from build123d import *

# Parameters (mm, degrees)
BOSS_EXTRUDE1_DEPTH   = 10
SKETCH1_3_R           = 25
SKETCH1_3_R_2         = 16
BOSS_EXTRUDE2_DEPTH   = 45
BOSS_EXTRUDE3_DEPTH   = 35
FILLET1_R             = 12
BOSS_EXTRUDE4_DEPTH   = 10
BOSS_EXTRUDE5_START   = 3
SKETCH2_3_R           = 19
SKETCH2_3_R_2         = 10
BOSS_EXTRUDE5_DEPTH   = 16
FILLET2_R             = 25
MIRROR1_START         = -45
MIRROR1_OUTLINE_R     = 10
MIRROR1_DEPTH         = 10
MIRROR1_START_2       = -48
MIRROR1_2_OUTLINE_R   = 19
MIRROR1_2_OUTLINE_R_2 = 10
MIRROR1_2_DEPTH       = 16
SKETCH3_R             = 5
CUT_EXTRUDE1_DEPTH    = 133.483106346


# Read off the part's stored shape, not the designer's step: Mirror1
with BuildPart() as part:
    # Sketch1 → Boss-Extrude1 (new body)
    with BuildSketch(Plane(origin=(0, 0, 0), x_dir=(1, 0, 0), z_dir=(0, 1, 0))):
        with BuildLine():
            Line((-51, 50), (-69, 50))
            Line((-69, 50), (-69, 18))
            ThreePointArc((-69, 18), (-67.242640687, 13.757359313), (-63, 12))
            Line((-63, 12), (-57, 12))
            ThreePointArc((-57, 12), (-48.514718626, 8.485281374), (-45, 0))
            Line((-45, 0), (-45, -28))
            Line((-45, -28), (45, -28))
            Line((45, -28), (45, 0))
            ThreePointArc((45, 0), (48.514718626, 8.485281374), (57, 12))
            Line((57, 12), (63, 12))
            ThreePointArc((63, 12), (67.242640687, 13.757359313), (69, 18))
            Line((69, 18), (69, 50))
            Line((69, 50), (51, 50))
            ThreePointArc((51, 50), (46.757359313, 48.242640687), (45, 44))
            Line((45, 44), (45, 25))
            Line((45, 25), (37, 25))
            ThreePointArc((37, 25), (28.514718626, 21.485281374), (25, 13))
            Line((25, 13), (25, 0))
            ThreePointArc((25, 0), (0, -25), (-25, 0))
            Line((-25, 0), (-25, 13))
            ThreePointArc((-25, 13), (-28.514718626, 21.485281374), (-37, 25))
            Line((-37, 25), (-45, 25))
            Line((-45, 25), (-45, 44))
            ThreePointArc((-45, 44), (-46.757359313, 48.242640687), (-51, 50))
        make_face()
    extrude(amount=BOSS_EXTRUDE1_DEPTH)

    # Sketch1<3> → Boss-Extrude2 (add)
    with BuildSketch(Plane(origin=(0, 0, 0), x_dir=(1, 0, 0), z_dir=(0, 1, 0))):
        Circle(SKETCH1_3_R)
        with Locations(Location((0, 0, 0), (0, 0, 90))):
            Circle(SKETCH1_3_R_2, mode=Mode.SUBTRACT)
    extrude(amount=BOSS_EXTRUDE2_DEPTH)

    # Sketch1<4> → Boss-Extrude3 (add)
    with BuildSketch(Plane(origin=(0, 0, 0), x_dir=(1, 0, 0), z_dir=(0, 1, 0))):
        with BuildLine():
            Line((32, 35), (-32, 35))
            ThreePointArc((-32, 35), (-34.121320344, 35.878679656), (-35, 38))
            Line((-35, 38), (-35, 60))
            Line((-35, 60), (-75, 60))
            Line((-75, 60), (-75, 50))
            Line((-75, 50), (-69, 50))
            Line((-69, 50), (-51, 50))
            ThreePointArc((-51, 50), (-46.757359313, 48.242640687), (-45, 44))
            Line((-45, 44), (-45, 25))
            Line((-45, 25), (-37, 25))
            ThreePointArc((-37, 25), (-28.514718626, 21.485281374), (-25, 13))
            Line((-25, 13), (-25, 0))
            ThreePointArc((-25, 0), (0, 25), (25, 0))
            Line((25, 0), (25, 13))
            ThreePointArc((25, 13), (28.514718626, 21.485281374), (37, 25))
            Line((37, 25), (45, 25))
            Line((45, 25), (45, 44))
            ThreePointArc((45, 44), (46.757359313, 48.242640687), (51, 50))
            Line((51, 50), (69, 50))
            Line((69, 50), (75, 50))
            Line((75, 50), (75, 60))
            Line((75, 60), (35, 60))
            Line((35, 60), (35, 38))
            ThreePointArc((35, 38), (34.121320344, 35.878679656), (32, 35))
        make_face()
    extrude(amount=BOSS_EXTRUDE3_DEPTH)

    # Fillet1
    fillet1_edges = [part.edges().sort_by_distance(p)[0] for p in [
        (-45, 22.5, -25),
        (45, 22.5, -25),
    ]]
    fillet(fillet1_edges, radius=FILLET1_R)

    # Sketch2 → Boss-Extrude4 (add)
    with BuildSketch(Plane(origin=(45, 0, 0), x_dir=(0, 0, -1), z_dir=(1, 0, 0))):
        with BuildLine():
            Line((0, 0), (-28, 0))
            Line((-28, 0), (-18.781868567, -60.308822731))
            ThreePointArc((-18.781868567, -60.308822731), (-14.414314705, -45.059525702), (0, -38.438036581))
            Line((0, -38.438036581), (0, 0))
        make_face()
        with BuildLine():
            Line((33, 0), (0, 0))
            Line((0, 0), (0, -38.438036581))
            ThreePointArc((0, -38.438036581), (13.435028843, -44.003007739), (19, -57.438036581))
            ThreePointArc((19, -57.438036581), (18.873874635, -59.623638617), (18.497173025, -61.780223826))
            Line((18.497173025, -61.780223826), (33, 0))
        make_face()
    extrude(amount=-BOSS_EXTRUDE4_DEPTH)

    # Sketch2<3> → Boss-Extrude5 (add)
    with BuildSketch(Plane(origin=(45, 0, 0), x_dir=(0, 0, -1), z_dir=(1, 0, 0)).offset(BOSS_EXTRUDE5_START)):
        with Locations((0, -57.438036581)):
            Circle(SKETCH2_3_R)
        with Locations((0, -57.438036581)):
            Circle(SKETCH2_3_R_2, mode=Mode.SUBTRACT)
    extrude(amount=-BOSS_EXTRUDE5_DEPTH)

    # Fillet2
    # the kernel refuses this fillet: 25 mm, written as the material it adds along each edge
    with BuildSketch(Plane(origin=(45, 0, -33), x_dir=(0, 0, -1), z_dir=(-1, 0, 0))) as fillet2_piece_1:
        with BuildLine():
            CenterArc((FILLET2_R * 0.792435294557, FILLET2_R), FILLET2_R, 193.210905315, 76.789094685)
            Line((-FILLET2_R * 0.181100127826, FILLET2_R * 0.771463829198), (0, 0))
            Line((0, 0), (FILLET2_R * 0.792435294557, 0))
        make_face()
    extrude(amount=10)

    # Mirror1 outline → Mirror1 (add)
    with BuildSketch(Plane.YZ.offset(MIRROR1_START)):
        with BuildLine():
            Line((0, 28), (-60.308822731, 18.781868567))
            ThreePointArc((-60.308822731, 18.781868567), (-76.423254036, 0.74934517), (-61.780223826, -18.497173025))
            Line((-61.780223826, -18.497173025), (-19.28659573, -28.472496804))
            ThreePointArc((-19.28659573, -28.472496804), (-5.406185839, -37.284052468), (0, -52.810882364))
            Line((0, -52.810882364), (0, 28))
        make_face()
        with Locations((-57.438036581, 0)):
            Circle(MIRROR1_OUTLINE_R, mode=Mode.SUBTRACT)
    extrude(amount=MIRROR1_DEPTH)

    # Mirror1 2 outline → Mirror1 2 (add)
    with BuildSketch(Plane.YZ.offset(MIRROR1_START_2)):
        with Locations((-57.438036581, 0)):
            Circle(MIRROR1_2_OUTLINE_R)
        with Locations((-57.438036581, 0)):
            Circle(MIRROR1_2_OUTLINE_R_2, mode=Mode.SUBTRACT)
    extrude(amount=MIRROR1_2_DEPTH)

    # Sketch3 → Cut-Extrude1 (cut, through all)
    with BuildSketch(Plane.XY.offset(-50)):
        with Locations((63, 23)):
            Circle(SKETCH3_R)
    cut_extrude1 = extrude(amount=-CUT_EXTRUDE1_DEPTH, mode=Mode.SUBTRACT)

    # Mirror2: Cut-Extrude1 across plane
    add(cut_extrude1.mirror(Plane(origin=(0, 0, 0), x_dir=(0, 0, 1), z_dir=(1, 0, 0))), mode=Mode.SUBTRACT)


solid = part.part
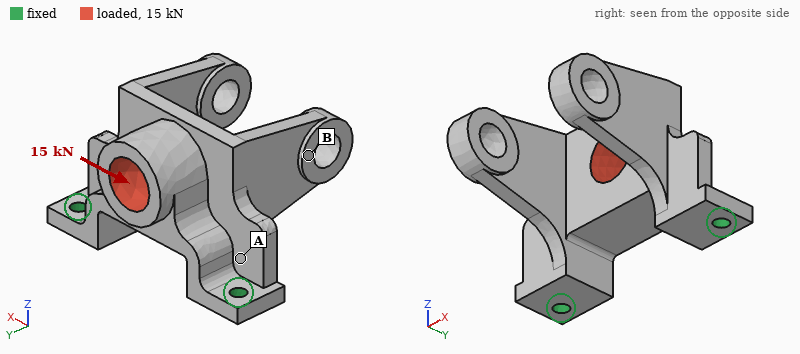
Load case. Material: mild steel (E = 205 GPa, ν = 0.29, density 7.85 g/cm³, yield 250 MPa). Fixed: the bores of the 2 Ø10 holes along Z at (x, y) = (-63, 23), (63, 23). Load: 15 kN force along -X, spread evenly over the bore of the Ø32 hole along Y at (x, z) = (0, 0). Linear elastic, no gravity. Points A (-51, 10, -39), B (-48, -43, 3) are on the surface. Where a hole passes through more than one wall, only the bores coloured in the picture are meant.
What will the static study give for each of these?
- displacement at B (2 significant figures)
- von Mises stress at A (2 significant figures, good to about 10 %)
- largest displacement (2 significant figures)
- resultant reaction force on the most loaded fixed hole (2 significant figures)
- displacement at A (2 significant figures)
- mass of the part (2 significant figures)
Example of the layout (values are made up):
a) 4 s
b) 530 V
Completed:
a) 22 µm
b) 40 MPa
c) 43 µm
d) 10 kN
e) 15 µm
f) 2.0 kg
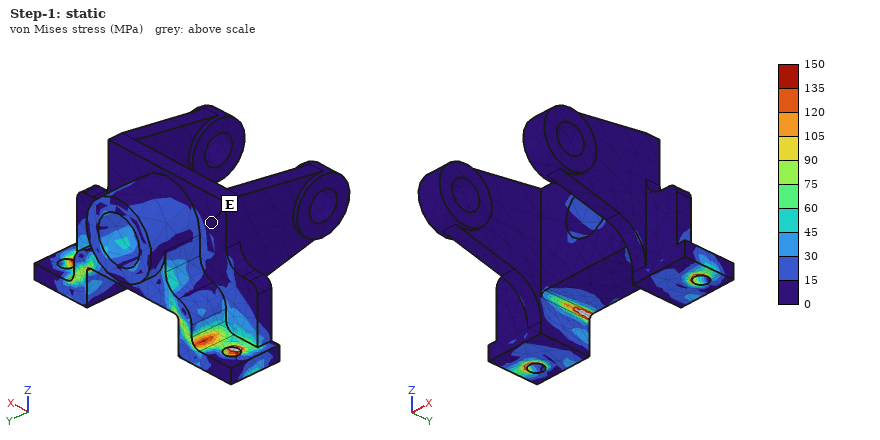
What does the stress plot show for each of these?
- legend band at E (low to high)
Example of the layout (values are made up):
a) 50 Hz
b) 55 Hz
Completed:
a) 0 to 15 MPa
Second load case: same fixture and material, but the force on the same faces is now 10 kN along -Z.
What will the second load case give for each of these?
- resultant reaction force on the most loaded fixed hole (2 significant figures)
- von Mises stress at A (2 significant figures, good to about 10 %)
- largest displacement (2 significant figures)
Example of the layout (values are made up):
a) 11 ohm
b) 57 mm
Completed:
a) 6.1 kN
b) 17 MPa
c) 45 µm
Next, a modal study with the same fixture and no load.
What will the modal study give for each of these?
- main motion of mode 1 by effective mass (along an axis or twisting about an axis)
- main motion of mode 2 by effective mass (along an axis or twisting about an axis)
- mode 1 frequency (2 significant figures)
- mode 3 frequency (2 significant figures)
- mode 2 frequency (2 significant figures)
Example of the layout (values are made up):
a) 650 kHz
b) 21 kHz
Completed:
a) along Y
b) along X
c) 690 Hz
d) 1300 Hz
e) 1200 Hz
